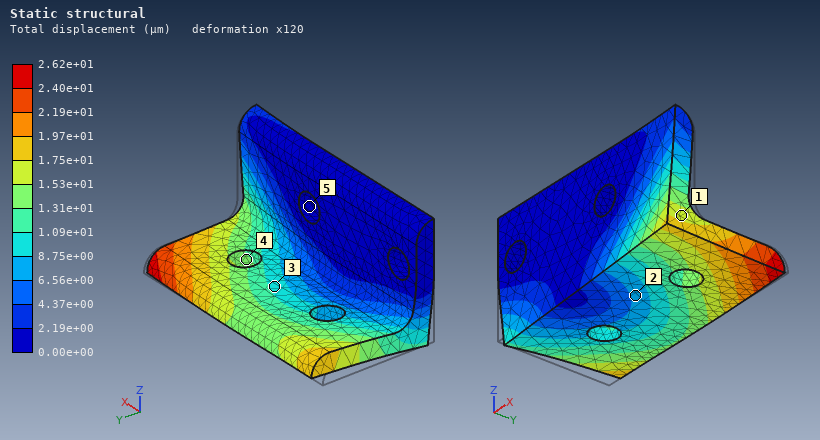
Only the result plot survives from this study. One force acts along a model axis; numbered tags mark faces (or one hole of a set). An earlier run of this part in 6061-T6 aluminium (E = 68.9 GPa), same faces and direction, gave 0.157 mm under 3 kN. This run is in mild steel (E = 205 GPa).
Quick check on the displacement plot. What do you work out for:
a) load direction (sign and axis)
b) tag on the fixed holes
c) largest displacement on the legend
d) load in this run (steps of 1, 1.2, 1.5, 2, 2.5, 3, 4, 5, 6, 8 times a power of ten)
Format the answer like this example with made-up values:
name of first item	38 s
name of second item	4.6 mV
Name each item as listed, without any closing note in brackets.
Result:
load direction	+X
tag on the fixed holes	5
largest displacement on the legend	2.62e+01 µm
load in this run	1.5 kN
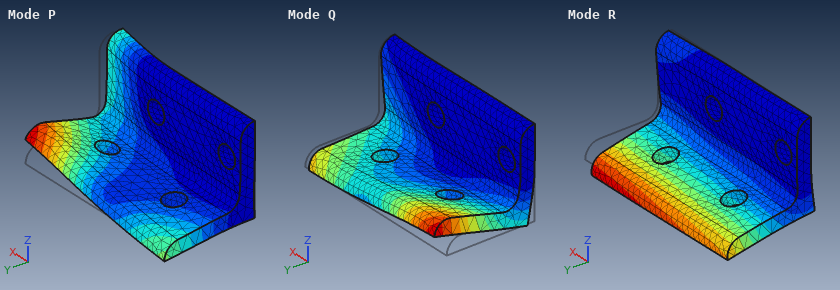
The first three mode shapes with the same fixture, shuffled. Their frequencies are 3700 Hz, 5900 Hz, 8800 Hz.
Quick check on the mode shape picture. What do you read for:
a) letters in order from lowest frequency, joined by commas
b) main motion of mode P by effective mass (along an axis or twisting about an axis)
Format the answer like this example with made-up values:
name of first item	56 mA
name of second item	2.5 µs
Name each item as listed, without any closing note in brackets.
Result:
letters in order from lowest frequency, joined by commas	R, Q, P
main motion of mode P by effective mass	along Y
